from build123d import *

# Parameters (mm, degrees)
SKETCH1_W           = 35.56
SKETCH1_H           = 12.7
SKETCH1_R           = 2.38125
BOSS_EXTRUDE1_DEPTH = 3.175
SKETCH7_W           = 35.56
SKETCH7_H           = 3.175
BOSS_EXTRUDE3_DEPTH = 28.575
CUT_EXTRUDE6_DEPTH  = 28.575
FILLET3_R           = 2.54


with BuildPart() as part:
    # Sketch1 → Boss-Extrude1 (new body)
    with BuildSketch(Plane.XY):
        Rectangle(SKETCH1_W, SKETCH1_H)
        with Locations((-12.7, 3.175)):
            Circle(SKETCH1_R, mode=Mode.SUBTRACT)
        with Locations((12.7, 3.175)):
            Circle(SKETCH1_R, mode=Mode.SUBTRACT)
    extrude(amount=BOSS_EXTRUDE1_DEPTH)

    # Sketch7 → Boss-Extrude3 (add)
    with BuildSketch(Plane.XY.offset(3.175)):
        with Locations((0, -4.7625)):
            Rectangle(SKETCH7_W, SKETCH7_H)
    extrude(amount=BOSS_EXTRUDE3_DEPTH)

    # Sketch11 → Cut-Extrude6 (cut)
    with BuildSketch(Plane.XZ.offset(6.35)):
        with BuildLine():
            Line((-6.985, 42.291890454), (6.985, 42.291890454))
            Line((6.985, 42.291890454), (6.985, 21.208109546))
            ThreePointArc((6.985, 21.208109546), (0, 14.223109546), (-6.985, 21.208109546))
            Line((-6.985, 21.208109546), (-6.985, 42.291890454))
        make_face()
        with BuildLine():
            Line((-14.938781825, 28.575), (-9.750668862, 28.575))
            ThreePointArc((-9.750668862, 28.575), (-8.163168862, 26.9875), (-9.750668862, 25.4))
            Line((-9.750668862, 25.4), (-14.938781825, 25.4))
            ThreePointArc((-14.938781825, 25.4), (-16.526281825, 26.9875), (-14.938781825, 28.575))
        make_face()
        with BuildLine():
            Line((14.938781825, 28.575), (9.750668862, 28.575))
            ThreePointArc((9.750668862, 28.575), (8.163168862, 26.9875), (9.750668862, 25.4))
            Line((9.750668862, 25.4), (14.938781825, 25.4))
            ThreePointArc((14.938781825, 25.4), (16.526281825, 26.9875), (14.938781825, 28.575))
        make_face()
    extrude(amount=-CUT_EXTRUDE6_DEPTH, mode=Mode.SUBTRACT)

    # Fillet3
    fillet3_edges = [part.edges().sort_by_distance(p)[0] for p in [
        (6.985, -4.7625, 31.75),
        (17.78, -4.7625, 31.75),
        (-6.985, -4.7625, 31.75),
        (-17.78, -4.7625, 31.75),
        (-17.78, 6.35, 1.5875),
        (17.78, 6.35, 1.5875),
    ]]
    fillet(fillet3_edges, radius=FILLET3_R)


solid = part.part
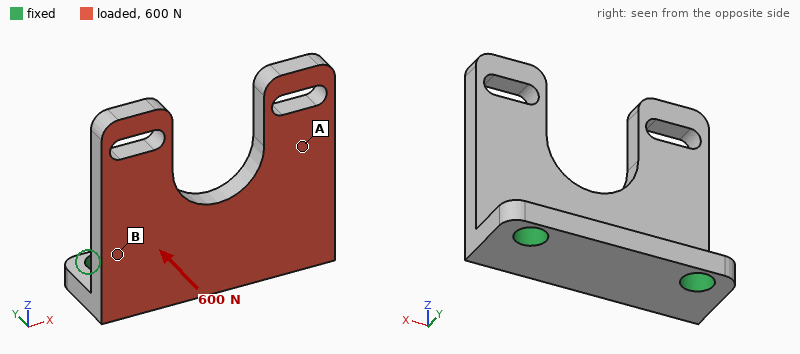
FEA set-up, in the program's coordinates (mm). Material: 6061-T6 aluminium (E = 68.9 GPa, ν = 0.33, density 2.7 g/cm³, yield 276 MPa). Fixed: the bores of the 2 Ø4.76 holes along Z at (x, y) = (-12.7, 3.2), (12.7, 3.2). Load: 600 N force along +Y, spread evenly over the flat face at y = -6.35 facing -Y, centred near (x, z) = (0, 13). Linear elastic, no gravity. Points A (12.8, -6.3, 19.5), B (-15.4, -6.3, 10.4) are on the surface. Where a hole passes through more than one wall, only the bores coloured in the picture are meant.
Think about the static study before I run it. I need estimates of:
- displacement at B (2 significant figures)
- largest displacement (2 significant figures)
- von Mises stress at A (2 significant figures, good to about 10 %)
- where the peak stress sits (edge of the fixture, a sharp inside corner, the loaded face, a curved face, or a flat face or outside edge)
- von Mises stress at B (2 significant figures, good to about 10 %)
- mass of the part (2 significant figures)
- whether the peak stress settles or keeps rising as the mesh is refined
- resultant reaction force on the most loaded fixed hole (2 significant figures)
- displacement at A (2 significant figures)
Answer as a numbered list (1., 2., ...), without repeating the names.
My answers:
1. 0.10 mm
2. 0.43 mm
3. 22 MPa
4. edge of the fixture
5. 56 MPa
6. 9.9 g
7. keeps rising
8. 310 N
9. 0.23 mm
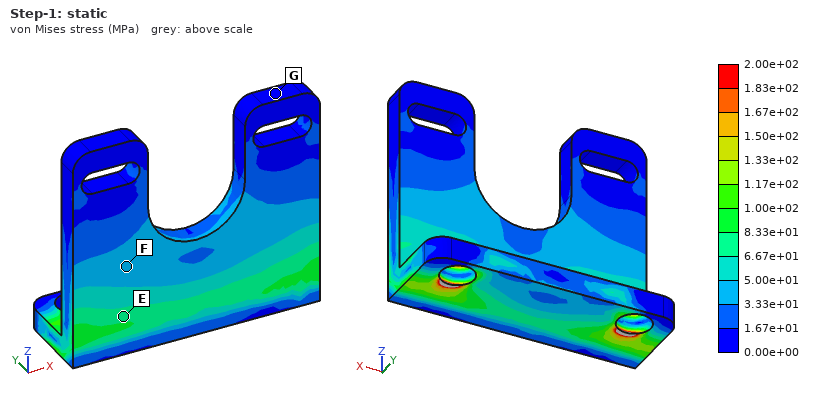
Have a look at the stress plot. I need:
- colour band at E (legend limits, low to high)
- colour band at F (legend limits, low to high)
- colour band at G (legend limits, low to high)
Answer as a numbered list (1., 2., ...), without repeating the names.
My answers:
1. 6.67e+01 to 8.33e+01 MPa
2. 3.33e+01 to 5.00e+01 MPa
3. 0.00e+00 to 1.67e+01 MPa
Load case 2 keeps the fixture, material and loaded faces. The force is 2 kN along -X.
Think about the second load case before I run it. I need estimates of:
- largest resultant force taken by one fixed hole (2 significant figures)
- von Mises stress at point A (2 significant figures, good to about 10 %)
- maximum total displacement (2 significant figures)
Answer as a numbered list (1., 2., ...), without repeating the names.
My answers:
1. 1.4 kN
2. 36 MPa
3. 0.11 mm
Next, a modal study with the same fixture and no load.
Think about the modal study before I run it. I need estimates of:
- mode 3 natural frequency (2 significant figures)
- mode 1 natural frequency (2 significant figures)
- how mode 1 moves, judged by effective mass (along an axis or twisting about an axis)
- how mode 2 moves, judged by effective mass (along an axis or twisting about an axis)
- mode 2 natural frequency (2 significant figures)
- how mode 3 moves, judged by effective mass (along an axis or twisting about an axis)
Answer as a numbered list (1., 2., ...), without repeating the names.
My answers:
1. 9500 Hz
2. 2900 Hz
3. along Y
4. twisting about Z
5. 4000 Hz
6. along X
